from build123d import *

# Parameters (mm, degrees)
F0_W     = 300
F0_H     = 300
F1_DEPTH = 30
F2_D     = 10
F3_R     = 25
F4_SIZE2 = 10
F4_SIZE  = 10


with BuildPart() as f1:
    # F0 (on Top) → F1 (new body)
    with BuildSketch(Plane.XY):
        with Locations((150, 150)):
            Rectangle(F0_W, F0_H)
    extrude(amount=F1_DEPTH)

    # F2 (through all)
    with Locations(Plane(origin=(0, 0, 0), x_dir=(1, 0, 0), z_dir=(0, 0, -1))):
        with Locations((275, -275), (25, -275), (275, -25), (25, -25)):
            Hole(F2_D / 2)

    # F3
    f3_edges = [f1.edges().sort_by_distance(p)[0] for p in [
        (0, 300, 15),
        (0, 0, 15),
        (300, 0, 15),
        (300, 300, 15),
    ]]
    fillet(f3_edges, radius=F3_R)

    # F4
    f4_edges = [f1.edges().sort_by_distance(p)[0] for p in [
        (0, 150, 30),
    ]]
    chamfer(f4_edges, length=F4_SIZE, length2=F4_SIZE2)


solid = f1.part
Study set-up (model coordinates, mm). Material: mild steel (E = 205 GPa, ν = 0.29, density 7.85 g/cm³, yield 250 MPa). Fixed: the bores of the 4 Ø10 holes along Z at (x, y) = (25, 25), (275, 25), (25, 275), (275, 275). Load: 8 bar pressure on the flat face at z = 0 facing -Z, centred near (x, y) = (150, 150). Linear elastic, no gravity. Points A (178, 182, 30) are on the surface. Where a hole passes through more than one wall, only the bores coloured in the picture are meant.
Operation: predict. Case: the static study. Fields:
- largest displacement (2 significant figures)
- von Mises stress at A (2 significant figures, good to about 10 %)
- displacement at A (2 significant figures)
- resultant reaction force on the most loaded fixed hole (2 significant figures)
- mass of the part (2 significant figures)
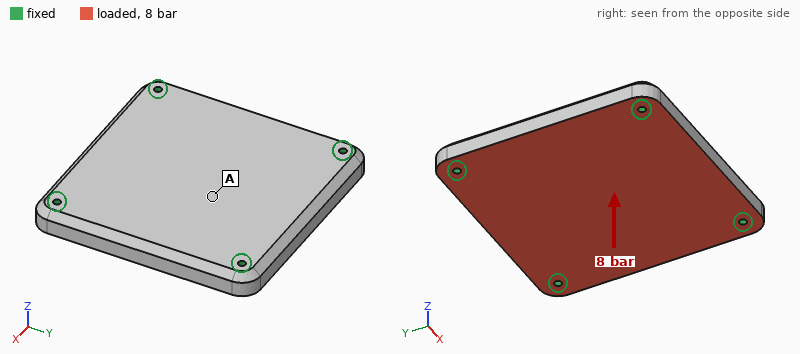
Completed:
67 µm
19 MPa
63 µm
18 kN
21 kg
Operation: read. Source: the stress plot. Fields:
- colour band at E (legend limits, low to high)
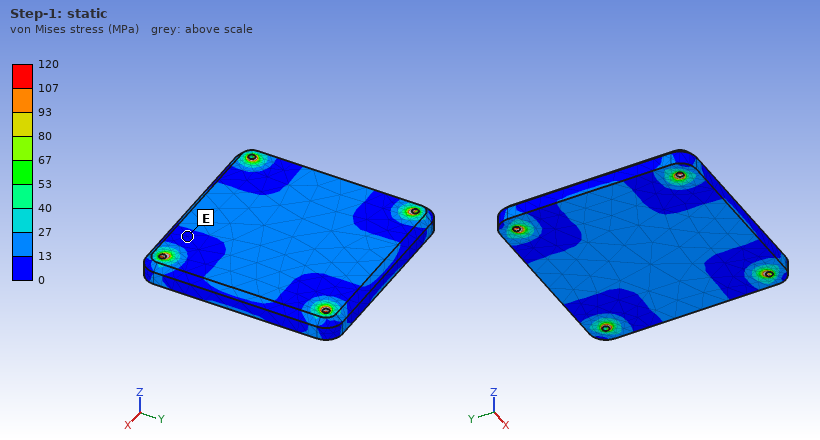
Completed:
0 to 13 MPa
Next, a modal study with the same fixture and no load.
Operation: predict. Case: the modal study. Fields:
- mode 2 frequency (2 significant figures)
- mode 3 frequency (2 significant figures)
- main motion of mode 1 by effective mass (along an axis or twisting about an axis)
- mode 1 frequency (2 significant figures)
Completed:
2300 Hz
2300 Hz
along Z
1400 Hz
